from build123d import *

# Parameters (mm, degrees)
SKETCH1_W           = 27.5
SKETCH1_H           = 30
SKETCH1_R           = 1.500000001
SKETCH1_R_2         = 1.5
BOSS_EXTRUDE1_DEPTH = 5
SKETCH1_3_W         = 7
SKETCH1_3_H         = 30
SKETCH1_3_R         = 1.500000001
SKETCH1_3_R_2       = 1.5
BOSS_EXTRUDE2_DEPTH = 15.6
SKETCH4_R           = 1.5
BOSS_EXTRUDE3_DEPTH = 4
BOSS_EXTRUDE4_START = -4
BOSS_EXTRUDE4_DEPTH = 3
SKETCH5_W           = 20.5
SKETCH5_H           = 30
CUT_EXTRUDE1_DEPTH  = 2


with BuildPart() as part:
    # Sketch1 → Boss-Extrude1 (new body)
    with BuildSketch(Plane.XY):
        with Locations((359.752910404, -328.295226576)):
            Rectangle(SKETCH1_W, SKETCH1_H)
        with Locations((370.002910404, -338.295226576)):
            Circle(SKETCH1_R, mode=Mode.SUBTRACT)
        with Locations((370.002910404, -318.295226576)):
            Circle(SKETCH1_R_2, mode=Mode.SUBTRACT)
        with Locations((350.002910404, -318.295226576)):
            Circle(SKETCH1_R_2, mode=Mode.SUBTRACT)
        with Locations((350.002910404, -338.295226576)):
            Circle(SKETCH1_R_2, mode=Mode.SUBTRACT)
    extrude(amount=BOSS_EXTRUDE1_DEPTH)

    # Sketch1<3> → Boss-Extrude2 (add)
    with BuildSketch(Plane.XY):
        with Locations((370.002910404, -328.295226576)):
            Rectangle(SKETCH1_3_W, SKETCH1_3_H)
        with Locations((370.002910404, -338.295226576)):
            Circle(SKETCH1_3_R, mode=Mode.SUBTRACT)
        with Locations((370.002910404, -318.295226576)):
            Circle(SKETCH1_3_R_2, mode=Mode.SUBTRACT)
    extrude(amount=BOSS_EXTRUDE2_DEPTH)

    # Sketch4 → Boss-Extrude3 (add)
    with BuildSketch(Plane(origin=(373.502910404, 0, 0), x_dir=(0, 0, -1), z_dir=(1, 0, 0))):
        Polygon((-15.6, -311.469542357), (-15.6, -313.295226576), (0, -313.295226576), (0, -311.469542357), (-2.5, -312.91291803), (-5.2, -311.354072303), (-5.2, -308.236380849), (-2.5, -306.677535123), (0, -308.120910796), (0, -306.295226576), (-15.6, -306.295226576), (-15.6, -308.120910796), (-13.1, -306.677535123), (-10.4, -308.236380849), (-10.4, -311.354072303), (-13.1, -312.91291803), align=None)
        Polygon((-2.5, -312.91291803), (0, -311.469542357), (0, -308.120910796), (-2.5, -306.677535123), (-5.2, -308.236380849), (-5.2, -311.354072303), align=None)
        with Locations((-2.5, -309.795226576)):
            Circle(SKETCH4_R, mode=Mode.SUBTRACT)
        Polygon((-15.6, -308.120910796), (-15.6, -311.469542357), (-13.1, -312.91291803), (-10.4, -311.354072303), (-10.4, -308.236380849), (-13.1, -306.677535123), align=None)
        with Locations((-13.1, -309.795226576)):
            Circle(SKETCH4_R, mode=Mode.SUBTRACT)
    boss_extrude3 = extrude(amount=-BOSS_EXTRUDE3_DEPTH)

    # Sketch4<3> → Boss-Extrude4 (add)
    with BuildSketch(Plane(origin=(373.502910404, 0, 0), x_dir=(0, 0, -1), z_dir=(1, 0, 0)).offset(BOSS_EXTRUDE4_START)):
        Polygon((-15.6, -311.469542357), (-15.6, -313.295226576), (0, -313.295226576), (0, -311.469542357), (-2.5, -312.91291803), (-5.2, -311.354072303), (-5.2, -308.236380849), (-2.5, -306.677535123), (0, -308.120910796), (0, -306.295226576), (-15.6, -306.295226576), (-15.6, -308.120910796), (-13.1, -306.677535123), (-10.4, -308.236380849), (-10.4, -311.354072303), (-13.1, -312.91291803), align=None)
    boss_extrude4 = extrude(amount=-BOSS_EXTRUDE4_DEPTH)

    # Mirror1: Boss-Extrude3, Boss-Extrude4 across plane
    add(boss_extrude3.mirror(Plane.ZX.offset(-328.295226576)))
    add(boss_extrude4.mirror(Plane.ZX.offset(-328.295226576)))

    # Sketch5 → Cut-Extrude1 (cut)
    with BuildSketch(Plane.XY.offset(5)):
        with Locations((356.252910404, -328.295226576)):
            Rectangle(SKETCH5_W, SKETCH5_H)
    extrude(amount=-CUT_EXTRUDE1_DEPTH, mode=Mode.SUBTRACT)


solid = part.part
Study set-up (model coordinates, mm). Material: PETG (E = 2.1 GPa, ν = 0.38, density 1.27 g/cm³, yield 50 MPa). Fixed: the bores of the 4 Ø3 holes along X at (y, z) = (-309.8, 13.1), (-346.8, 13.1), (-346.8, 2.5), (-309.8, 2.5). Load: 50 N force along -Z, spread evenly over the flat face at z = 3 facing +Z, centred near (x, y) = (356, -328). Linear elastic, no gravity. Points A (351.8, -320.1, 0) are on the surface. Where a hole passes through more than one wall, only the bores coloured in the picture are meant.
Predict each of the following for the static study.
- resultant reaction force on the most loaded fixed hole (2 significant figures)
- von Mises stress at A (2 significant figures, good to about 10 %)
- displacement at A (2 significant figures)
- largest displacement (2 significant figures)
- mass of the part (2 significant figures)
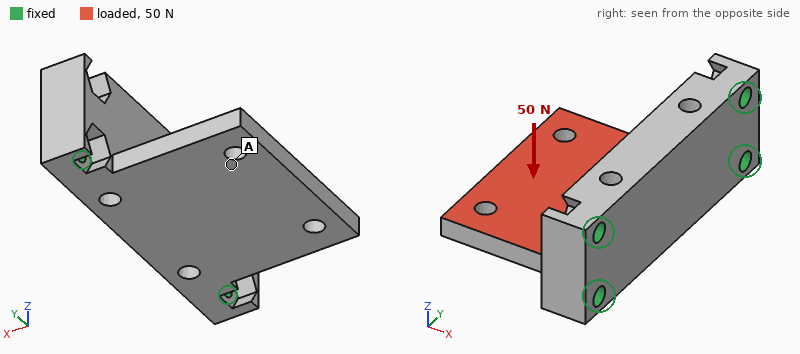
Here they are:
43 N
1.3 MPa
0.37 mm
0.56 mm
7.6 g
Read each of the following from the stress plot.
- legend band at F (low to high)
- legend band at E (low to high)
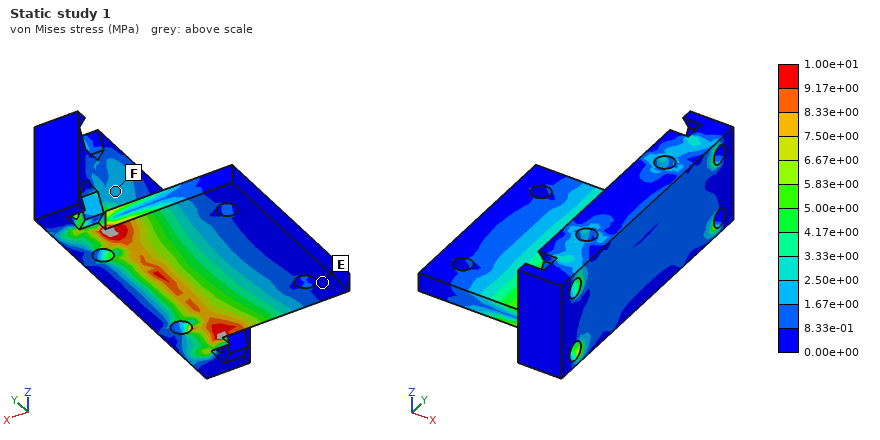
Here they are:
1.67e+00 to 2.50e+00 MPa
0.00e+00 to 8.33e-01 MPa
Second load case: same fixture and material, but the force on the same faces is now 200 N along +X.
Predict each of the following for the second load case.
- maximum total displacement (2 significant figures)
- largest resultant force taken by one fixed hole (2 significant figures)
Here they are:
0.28 mm
100 N
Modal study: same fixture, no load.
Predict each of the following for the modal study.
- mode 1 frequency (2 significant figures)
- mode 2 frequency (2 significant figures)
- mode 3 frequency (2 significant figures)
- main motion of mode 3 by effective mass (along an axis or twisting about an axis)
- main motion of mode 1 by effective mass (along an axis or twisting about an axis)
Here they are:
1200 Hz
2400 Hz
4700 Hz
along X
along Z
